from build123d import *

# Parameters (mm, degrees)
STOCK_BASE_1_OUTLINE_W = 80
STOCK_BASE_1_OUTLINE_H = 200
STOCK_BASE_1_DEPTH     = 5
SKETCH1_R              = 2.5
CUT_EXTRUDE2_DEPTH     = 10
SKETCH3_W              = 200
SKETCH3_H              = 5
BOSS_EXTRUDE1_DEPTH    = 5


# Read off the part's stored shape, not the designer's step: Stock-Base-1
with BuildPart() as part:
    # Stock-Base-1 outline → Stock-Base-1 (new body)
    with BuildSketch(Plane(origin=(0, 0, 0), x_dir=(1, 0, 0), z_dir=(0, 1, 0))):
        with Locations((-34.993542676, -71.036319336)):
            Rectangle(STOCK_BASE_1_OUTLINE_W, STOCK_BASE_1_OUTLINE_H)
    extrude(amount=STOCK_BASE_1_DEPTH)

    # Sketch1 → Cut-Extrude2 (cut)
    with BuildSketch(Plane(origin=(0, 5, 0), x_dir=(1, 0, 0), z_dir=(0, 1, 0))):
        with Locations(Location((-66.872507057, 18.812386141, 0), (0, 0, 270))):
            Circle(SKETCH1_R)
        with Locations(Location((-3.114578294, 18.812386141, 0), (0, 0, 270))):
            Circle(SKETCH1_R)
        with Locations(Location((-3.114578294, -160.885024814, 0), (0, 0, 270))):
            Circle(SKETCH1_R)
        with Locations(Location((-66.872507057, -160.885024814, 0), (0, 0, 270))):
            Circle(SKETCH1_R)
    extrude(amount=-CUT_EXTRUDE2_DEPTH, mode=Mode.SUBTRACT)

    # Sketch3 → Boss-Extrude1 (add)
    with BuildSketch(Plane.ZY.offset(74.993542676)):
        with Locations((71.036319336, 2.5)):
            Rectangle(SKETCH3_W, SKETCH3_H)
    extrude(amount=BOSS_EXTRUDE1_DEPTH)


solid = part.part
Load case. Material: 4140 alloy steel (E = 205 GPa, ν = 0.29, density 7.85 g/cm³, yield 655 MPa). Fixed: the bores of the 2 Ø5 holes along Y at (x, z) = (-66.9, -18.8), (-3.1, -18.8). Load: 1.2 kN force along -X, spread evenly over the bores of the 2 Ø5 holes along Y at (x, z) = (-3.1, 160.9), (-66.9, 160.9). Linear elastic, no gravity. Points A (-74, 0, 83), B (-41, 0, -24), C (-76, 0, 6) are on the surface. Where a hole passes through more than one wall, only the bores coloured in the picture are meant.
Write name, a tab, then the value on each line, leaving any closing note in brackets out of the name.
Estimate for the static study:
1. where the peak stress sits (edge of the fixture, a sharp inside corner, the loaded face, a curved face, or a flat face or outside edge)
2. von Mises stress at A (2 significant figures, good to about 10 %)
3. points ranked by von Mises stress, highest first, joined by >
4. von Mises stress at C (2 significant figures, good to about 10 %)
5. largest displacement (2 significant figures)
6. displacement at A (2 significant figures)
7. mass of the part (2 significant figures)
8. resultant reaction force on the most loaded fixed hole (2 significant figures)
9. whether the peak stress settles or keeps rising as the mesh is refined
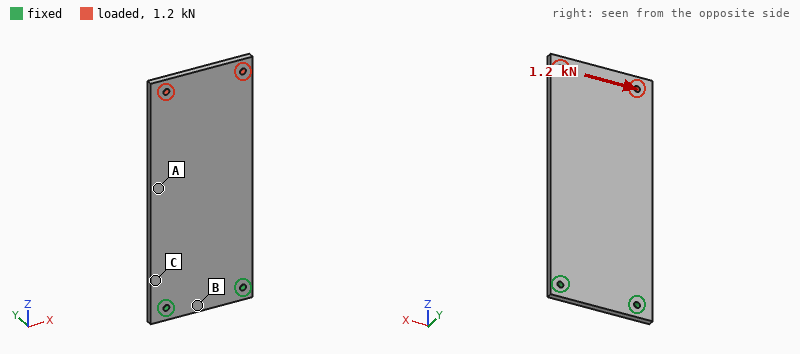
where the peak stress sits	edge of the fixture
von Mises stress at A	13 MPa
points ranked by von Mises stress, highest first, joined by >	C > A > B
von Mises stress at C	26 MPa
largest displacement	63 µm
displacement at A	27 µm
mass of the part	660 g
resultant reaction force on the most loaded fixed hole	3.4 kN
whether the peak stress settles or keeps rising as the mesh is refined	keeps rising
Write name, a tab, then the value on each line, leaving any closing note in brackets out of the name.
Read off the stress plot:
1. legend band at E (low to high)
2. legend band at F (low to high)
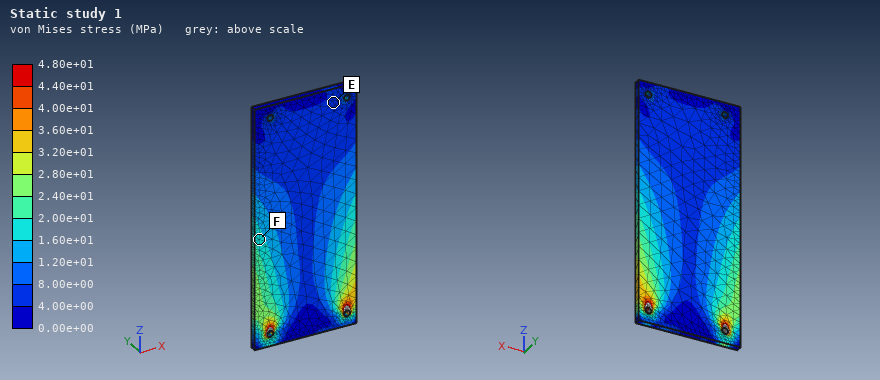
legend band at E	4.00e+00 to 8.00e+00 MPa
legend band at F	1.60e+01 to 2.00e+01 MPa
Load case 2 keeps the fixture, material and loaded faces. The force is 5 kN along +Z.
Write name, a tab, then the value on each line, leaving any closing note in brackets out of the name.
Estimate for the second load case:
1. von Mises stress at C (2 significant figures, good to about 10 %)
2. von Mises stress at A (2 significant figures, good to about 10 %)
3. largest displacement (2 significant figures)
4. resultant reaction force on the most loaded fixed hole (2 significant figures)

von Mises stress at C	13 MPa
von Mises stress at A	10 MPa
largest displacement	17 µm
resultant reaction force on the most loaded fixed hole	2.6 kN
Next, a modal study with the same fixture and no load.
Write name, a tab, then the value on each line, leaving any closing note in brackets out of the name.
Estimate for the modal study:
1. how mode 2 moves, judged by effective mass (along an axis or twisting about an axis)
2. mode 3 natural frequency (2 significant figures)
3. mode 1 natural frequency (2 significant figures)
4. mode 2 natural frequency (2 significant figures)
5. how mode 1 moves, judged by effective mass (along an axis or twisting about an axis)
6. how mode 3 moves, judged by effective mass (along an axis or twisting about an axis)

how mode 2 moves, judged by effective mass	twisting about Z
mode 3 natural frequency	690 Hz
mode 1 natural frequency	110 Hz
mode 2 natural frequency	550 Hz
how mode 1 moves, judged by effective mass	along Y
how mode 3 moves, judged by effective mass	along Y
